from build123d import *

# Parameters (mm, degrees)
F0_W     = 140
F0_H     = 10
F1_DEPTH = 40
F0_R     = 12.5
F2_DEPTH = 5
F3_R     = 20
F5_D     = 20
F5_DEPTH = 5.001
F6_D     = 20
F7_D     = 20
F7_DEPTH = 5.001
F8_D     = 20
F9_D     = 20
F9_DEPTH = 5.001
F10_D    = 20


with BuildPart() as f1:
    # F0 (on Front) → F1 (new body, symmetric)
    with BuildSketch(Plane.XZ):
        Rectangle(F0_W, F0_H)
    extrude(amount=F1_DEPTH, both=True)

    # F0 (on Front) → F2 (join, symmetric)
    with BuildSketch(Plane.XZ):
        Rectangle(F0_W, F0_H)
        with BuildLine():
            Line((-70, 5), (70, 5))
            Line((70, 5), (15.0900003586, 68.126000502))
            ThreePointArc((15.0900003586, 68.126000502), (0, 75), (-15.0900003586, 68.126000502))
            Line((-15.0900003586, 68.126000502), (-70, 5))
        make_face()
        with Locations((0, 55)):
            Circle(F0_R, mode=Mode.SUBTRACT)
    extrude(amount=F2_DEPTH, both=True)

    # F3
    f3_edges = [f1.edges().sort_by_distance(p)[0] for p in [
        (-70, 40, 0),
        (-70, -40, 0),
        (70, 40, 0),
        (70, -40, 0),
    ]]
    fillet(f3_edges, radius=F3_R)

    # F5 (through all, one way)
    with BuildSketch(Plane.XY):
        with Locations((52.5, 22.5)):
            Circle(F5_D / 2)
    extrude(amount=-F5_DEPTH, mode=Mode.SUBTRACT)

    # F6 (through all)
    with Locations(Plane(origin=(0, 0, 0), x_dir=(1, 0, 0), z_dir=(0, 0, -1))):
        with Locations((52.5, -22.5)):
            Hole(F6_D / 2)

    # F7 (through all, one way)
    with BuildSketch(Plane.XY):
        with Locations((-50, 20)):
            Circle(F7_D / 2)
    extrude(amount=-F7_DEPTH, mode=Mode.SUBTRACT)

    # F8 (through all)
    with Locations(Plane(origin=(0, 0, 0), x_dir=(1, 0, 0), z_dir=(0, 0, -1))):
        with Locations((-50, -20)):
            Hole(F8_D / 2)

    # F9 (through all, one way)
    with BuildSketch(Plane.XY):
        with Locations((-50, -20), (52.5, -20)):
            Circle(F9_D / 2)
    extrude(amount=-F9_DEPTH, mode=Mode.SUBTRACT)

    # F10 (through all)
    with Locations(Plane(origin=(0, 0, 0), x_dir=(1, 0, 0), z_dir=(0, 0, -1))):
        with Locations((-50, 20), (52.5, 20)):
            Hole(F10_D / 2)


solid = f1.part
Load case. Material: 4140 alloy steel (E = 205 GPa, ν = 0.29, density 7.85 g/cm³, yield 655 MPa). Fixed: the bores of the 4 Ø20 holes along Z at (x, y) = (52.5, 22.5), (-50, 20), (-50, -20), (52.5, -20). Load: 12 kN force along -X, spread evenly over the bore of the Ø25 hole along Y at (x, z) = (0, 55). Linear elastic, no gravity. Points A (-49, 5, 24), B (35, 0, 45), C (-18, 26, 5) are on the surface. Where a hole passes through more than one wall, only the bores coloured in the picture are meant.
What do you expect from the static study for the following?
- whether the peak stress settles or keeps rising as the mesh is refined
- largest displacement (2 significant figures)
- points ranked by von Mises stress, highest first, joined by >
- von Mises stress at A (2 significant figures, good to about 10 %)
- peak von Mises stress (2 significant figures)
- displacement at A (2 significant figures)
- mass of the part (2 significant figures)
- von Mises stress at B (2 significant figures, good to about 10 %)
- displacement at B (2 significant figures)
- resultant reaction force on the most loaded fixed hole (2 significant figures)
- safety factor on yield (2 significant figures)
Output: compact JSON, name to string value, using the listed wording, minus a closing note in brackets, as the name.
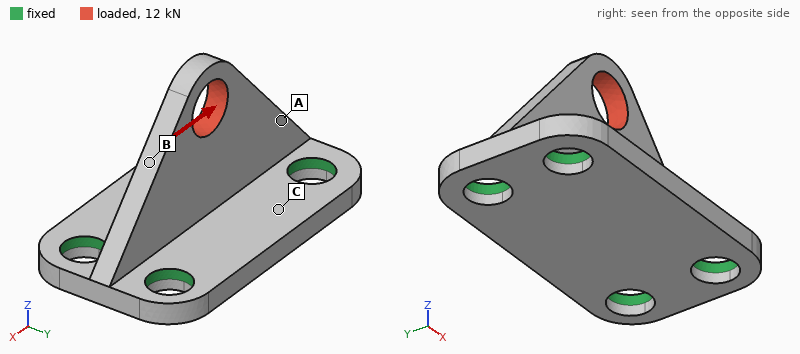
{"whether the peak stress settles or keeps rising as the mesh is refined": "settles", "largest displacement": "30 µm", "points ranked by von Mises stress, highest first, joined by >": "B > A > C", "von Mises stress at A": "28 MPa", "peak von Mises stress": "100 MPa", "displacement at A": "5.9 µm", "mass of the part": "1.1 kg", "von Mises stress at B": "50 MPa", "displacement at B": "12 µm", "resultant reaction force on the most loaded fixed hole": "4.7 kN", "safety factor on yield": "6.4"}
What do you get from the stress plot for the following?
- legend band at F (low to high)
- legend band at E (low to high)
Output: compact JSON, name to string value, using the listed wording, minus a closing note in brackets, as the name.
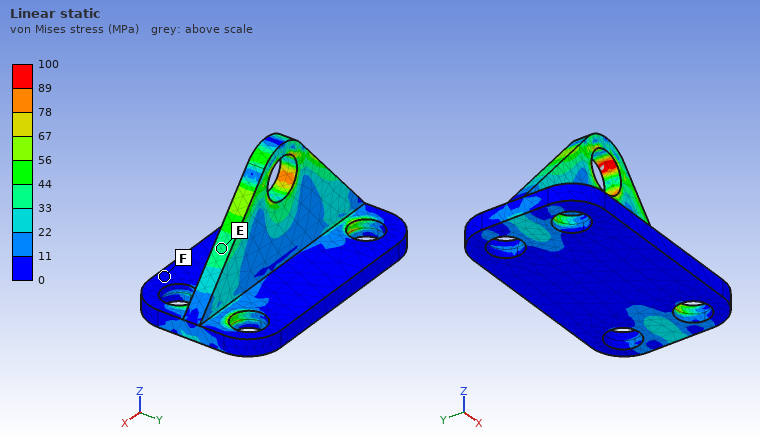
{"legend band at F": "0 to 11 MPa", "legend band at E": "33 to 44 MPa"}
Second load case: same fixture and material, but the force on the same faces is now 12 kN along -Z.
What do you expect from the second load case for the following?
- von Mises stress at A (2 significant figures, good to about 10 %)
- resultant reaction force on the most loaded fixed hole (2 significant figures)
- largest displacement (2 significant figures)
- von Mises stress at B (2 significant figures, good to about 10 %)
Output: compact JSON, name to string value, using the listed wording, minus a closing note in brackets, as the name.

{"von Mises stress at A": "15 MPa", "resultant reaction force on the most loaded fixed hole": "3.4 kN", "largest displacement": "15 µm", "von Mises stress at B": "20 MPa"}
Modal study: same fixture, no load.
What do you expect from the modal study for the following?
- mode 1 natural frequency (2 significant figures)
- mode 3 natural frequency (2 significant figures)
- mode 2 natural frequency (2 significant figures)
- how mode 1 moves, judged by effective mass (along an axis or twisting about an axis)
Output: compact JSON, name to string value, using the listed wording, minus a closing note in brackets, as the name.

{"mode 1 natural frequency": "2500 Hz", "mode 3 natural frequency": "6800 Hz", "mode 2 natural frequency": "6000 Hz", "how mode 1 moves, judged by effective mass": "along Y"}
